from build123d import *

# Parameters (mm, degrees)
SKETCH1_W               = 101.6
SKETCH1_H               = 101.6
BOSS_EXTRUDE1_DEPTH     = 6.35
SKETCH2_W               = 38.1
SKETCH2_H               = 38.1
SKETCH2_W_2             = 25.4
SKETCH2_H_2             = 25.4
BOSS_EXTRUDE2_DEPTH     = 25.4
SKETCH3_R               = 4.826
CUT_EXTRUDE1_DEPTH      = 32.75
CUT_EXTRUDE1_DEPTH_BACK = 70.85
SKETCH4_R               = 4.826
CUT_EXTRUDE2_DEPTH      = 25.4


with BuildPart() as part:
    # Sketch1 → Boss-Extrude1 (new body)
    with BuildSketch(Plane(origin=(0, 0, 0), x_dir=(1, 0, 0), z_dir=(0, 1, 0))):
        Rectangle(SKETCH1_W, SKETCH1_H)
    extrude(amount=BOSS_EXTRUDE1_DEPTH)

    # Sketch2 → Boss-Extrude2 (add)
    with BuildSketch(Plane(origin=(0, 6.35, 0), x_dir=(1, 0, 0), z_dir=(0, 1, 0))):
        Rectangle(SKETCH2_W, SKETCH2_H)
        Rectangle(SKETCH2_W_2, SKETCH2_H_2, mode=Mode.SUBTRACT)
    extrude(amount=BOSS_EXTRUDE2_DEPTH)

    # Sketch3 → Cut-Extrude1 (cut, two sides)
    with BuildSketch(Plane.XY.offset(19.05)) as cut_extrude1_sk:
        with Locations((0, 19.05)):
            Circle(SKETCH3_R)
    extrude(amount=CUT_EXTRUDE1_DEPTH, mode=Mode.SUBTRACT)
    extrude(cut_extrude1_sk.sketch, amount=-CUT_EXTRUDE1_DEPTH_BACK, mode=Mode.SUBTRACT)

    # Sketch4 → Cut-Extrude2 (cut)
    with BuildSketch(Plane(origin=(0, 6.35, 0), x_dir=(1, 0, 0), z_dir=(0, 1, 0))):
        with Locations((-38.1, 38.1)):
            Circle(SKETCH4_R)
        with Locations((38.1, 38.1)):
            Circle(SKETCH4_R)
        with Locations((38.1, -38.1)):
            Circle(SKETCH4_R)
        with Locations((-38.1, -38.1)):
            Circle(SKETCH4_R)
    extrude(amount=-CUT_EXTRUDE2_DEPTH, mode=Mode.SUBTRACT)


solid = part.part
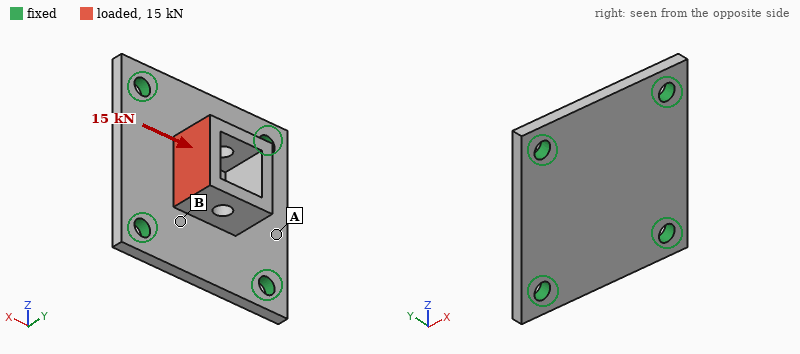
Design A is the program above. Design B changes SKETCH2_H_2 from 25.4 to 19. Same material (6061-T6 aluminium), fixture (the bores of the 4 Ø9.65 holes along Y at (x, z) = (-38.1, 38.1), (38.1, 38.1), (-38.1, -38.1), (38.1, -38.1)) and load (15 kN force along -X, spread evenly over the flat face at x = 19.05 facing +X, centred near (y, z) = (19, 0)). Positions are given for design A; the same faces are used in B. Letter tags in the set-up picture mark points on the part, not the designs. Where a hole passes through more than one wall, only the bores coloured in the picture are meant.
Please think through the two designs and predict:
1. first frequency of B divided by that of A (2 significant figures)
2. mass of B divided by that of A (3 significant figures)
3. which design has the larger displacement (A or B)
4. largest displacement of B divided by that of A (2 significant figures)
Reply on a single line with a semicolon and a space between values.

0.97; 1.04; A; 0.83
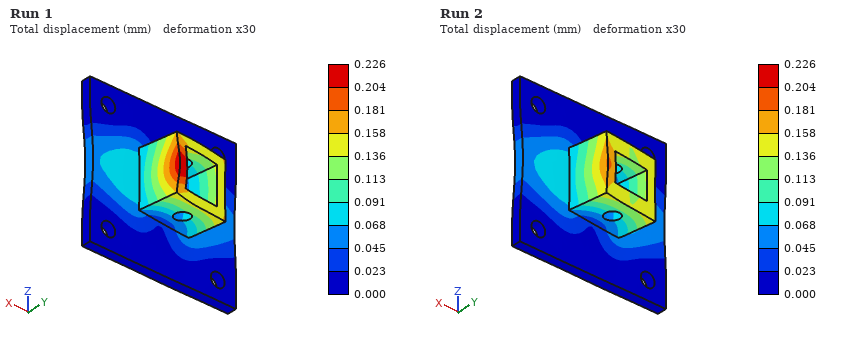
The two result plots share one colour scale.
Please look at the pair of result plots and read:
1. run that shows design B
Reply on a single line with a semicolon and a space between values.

Run 2
